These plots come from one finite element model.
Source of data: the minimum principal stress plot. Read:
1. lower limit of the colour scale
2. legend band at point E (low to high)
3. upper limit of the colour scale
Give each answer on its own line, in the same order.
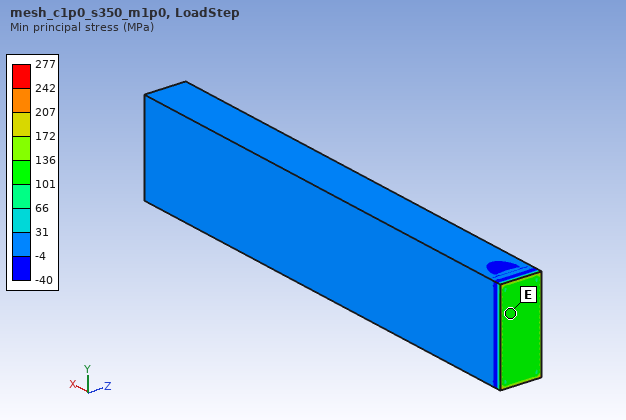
-40 MPa
101 to 136 MPa
277 MPa
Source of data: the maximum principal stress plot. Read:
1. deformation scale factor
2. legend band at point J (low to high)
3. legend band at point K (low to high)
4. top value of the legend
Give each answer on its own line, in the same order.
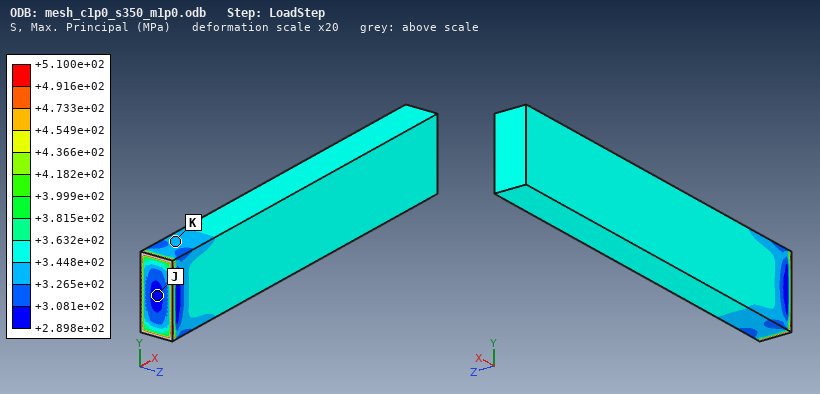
20
+2.898e+02 to +3.081e+02 MPa
+3.265e+02 to +3.448e+02 MPa
+5.100e+02 MPa
